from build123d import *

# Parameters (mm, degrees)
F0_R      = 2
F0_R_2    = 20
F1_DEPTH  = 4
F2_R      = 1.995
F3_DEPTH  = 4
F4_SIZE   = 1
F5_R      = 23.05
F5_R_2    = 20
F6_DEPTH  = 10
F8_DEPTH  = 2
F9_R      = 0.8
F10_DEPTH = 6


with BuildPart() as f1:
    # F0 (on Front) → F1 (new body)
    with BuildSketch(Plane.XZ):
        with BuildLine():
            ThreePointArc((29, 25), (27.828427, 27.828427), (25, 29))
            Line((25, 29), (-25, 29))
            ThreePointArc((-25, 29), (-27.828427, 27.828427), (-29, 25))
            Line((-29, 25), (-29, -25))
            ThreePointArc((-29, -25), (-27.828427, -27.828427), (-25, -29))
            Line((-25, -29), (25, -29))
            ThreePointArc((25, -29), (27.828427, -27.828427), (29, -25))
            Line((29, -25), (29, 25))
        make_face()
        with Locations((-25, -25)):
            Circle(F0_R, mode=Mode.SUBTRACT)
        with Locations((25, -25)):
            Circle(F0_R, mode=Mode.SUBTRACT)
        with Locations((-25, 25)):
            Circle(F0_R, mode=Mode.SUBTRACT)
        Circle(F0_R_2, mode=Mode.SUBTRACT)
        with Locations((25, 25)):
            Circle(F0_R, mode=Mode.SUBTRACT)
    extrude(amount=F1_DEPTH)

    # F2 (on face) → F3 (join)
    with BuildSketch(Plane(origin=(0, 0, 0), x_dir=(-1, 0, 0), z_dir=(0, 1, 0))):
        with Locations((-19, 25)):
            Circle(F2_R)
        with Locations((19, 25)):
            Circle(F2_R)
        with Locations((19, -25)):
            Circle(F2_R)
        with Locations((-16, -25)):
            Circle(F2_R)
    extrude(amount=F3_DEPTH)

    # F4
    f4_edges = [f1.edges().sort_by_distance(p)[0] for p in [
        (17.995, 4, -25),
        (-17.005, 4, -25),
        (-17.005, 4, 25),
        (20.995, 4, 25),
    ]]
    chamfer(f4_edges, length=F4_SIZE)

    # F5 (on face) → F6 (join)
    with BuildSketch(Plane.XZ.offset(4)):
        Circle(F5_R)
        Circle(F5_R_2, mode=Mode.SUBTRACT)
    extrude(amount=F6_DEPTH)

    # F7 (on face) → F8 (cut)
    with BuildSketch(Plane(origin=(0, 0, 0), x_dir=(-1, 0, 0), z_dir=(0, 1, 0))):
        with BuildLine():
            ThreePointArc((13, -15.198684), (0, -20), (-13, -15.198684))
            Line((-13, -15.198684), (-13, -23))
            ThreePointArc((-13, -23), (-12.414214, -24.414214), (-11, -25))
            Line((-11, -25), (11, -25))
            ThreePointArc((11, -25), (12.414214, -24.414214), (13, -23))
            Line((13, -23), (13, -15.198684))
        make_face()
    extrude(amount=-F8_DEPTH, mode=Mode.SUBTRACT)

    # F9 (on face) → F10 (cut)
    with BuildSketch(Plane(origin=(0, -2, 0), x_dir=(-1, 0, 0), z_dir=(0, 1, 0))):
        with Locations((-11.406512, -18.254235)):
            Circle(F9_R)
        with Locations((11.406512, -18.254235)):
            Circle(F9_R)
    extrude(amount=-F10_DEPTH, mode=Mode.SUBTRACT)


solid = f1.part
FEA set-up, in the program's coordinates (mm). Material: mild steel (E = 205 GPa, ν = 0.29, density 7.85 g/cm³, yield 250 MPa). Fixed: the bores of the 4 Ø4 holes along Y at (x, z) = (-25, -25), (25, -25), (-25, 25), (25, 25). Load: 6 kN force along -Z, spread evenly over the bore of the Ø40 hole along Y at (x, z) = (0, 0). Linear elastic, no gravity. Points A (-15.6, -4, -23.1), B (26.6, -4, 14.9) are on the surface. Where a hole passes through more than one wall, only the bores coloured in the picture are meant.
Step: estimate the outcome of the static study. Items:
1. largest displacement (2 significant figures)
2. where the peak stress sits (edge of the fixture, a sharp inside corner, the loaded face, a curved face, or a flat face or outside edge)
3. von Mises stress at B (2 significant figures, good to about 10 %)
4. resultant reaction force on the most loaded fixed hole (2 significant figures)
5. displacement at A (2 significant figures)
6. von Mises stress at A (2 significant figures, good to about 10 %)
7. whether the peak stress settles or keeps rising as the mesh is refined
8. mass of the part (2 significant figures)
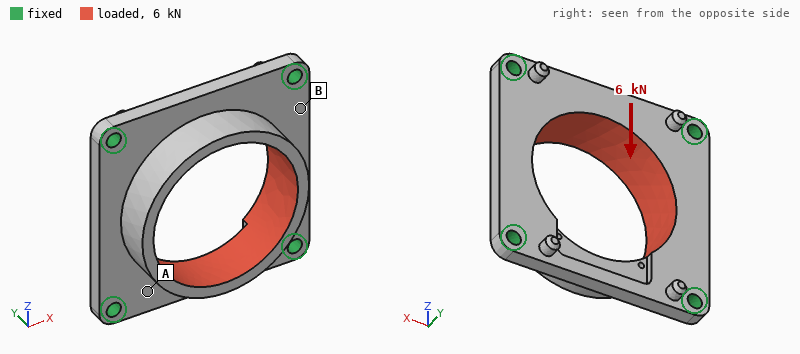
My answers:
18 µm
edge of the fixture
41 MPa
1.6 kN
5.2 µm
25 MPa
keeps rising
95 g
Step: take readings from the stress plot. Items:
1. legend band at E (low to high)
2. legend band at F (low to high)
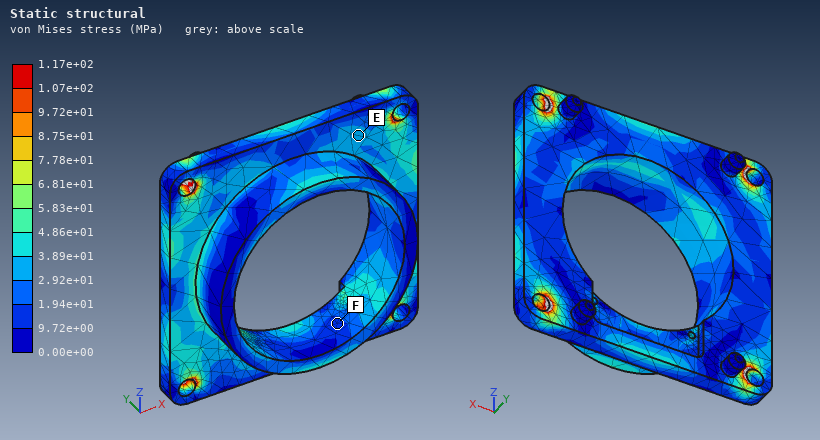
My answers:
2.92e+01 to 3.89e+01 MPa
9.72e+00 to 1.94e+01 MPa
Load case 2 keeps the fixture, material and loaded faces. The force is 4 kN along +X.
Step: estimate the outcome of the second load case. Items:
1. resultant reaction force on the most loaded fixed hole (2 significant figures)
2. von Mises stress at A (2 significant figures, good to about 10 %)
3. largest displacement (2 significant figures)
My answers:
1.1 kN
23 MPa
11 µm
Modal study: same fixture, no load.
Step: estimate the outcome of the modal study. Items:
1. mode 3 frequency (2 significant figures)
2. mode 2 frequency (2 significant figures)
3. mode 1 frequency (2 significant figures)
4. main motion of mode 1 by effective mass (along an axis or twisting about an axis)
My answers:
9500 Hz
9500 Hz
8300 Hz
along Y
